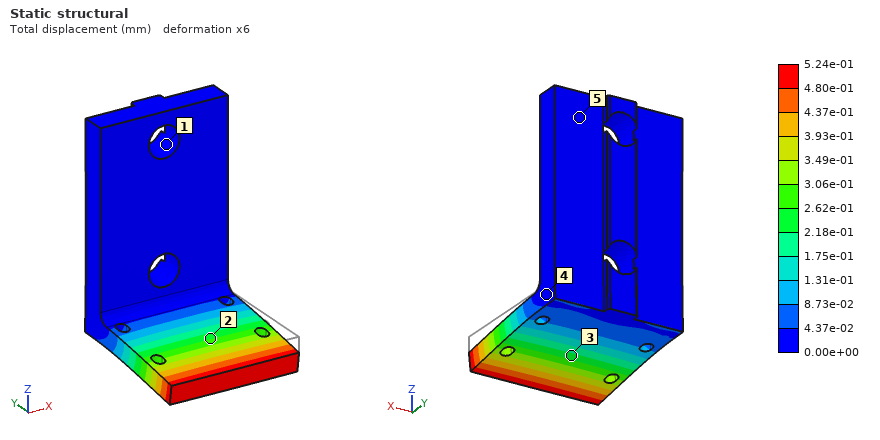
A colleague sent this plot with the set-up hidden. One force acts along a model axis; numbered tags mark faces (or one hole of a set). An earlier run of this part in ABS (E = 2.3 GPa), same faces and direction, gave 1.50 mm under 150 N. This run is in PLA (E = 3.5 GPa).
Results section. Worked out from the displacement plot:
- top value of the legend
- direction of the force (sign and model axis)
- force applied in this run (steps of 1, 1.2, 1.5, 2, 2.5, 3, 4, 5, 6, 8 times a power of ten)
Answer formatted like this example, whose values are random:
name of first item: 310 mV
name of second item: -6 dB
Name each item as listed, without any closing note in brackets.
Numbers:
top value of the legend: 5.24e-01 mm
direction of the force: -Z
force applied in this run: 80 N
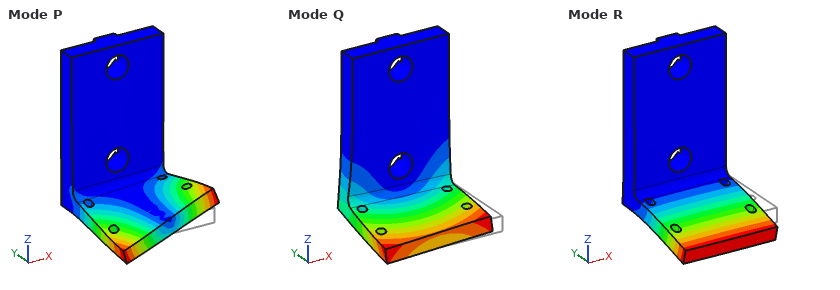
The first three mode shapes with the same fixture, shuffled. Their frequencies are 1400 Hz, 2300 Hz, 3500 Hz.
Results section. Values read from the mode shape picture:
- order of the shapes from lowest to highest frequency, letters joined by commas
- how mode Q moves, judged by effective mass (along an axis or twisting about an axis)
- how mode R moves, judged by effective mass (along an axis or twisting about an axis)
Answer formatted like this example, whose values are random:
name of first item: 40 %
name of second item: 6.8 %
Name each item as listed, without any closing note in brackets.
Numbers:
order of the shapes from lowest to highest frequency, letters joined by commas: R, Q, P
how mode Q moves, judged by effective mass: along X
how mode R moves, judged by effective mass: along Z
